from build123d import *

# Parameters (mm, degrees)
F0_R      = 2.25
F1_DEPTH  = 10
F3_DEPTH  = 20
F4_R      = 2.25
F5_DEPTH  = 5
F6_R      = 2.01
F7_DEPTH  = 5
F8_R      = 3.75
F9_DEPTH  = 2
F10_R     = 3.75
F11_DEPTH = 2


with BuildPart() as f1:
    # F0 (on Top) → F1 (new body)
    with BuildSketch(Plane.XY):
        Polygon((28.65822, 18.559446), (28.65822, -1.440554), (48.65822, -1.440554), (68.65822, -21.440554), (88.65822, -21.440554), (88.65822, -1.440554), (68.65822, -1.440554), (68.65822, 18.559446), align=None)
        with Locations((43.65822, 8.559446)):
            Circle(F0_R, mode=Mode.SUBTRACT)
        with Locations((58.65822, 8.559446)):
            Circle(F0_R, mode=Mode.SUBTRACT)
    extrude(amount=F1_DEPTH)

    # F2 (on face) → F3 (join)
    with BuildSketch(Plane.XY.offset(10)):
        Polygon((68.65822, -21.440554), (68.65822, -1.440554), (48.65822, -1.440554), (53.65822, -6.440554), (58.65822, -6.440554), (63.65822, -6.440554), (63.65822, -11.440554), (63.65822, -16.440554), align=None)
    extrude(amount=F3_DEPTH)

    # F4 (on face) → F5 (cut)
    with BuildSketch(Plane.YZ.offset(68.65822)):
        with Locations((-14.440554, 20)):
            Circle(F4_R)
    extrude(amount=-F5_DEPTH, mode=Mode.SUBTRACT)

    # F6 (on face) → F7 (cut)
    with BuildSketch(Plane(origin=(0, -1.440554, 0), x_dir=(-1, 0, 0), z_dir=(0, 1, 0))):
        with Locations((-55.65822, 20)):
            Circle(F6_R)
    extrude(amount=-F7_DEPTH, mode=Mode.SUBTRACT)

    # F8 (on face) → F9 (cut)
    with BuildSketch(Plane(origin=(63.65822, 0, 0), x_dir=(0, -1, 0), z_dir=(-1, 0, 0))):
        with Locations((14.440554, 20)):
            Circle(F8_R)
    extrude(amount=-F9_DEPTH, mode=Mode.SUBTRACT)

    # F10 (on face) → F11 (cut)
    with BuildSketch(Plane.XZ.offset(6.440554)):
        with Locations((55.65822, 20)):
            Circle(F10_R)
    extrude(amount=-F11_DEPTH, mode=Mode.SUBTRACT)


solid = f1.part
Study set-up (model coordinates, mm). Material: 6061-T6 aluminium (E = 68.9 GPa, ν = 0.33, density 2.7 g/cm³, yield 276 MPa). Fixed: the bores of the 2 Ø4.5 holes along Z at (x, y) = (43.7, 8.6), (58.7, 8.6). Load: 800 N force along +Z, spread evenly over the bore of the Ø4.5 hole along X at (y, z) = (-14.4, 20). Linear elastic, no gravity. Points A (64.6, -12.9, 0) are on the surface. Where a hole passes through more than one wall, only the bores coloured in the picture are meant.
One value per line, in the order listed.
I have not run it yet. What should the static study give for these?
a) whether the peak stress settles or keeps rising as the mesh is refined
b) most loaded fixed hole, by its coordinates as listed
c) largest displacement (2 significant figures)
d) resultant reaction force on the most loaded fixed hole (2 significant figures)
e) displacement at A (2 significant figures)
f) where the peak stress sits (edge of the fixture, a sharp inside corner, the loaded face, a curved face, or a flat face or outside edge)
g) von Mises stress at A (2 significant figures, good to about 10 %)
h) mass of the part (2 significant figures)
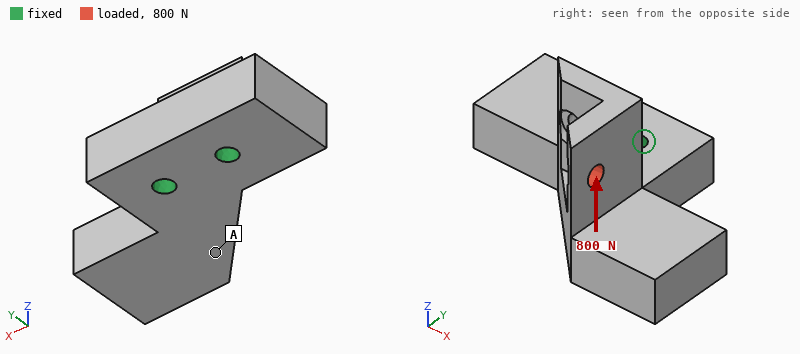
keeps rising
(58.7, 8.6)
80 µm
910 N
35 µm
edge of the fixture
8.4 MPa
44 g
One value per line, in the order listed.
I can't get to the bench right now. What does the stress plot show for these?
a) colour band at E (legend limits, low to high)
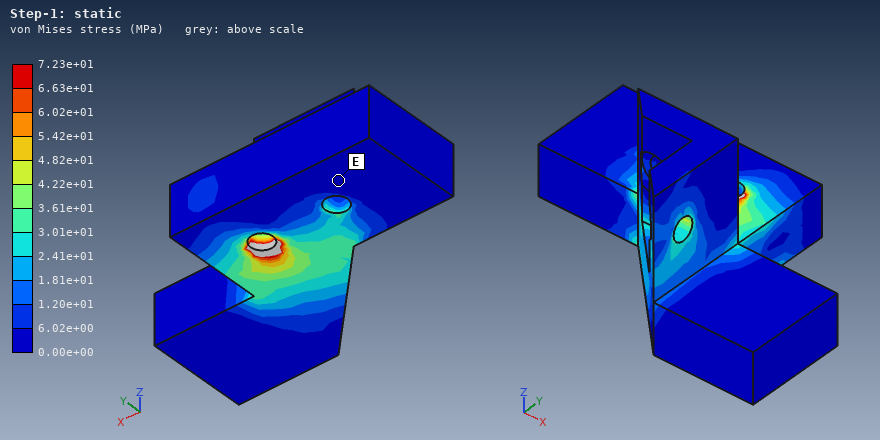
0.00e+00 to 6.02e+00 MPa
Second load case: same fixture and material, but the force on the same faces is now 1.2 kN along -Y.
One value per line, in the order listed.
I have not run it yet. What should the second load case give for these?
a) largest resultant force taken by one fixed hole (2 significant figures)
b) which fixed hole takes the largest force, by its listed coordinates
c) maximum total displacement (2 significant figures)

1.7 kN
(58.7, 8.6)
0.12 mm
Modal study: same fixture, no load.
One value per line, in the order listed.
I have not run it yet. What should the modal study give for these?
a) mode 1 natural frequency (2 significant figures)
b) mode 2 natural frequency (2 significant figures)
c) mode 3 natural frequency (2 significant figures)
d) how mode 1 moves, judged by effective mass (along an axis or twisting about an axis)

4400 Hz
6800 Hz
8000 Hz
along Z
